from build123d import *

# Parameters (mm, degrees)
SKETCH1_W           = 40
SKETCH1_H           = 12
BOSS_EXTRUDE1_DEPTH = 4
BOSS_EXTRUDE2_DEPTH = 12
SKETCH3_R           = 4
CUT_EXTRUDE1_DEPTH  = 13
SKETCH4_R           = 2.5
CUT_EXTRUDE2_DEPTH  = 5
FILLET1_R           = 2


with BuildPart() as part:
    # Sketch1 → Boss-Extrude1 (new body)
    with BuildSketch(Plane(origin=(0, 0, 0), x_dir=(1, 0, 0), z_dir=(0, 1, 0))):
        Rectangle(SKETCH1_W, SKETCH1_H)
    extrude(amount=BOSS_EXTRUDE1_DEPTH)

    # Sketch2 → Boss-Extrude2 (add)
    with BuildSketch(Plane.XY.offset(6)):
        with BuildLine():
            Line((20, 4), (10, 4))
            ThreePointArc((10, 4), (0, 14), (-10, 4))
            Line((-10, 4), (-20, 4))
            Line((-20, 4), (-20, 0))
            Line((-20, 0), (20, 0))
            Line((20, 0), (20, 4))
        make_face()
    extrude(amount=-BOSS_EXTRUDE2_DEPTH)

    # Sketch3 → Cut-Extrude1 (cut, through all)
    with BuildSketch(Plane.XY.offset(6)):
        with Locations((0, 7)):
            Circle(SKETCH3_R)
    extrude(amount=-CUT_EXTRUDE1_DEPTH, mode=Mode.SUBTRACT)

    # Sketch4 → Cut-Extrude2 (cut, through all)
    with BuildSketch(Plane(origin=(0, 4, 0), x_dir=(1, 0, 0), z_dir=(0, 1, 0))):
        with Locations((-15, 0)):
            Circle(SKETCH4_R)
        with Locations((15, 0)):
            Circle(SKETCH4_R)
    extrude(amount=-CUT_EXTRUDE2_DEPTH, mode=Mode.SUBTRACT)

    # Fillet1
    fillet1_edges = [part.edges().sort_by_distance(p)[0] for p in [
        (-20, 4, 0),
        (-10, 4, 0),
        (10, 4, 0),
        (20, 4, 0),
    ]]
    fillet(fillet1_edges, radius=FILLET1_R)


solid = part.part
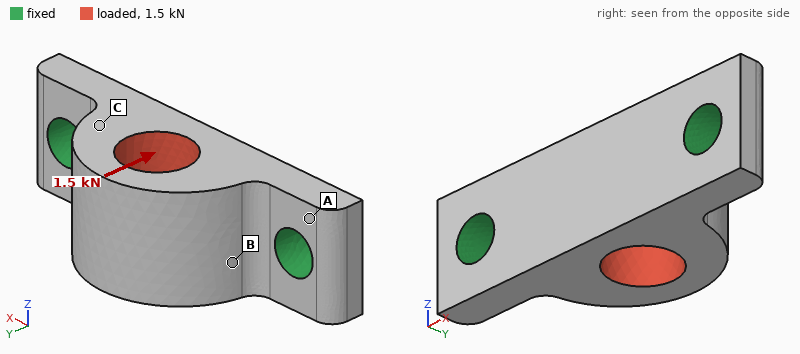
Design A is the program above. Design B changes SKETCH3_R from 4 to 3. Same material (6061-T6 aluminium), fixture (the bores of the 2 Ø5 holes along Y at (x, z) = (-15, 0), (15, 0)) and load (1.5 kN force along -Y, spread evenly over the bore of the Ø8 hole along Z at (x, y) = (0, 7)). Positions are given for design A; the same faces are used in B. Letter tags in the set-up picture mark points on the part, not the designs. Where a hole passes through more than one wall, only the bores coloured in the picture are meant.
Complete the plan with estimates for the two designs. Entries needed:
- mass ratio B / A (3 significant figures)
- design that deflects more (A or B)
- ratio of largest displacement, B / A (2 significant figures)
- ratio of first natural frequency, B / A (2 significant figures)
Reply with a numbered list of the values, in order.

1. 1.09
2. A
3. 0.86
4. 0.95
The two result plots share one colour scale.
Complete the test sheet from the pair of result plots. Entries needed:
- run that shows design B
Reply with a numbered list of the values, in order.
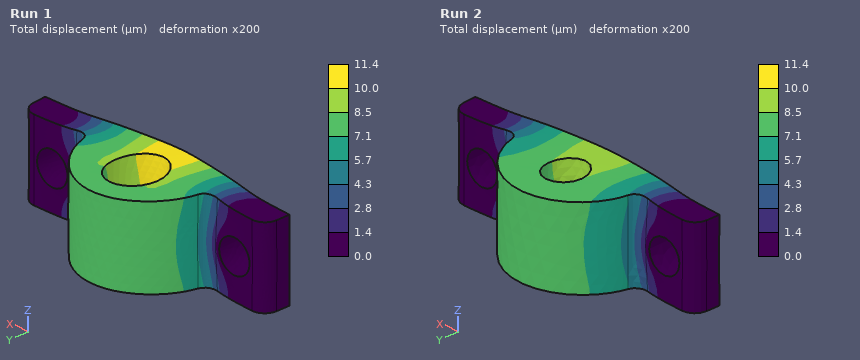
1. Run 2
